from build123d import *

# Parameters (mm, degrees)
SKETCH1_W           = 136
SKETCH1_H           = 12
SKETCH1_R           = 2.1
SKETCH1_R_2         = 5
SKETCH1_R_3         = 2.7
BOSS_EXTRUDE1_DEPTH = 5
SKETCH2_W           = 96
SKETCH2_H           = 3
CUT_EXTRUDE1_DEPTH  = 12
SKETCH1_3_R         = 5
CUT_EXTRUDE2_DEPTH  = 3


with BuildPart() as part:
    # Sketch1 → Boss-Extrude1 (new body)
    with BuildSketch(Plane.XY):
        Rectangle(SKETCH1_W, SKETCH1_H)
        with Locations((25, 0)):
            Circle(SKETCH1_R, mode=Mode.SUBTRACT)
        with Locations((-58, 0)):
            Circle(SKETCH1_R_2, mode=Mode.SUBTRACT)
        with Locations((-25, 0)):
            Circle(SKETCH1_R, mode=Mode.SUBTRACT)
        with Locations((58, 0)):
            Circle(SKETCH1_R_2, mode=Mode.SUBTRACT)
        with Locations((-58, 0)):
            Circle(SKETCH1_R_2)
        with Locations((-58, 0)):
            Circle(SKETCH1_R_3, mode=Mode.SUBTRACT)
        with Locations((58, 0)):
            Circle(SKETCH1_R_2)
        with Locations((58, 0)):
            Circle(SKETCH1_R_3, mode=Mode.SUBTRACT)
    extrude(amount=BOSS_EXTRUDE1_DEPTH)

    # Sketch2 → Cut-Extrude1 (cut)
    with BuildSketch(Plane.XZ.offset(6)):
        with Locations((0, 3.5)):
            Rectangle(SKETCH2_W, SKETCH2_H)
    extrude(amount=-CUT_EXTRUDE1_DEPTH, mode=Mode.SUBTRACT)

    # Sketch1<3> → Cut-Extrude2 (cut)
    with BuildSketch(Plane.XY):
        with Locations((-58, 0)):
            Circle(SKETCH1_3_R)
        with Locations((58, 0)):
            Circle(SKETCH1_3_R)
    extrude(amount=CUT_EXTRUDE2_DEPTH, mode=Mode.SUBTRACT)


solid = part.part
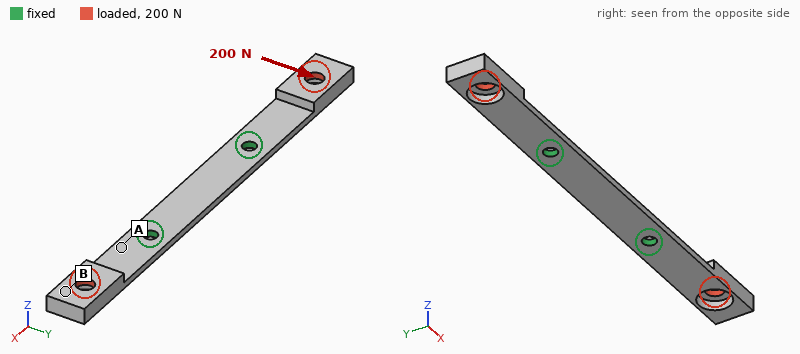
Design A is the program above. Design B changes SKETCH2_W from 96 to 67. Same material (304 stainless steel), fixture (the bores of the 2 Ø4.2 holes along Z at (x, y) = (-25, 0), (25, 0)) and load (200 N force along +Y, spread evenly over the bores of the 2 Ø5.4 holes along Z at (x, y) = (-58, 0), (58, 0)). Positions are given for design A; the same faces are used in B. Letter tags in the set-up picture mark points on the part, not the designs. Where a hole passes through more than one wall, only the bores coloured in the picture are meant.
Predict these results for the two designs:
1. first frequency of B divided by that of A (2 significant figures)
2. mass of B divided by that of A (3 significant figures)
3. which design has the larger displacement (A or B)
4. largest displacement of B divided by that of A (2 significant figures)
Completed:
1.2
1.26
A
0.70
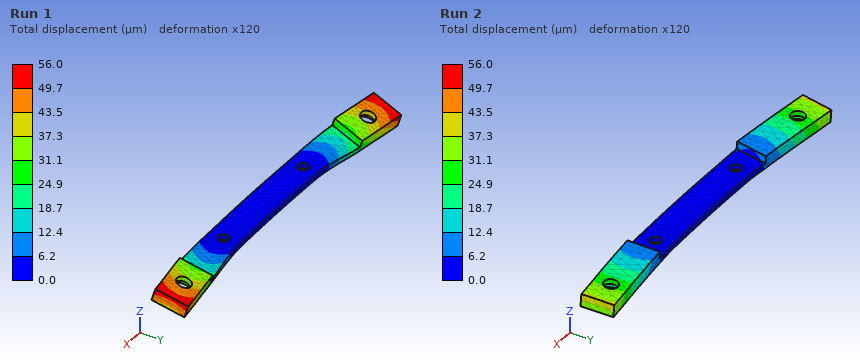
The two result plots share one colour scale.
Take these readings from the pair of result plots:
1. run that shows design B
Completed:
Run 2
